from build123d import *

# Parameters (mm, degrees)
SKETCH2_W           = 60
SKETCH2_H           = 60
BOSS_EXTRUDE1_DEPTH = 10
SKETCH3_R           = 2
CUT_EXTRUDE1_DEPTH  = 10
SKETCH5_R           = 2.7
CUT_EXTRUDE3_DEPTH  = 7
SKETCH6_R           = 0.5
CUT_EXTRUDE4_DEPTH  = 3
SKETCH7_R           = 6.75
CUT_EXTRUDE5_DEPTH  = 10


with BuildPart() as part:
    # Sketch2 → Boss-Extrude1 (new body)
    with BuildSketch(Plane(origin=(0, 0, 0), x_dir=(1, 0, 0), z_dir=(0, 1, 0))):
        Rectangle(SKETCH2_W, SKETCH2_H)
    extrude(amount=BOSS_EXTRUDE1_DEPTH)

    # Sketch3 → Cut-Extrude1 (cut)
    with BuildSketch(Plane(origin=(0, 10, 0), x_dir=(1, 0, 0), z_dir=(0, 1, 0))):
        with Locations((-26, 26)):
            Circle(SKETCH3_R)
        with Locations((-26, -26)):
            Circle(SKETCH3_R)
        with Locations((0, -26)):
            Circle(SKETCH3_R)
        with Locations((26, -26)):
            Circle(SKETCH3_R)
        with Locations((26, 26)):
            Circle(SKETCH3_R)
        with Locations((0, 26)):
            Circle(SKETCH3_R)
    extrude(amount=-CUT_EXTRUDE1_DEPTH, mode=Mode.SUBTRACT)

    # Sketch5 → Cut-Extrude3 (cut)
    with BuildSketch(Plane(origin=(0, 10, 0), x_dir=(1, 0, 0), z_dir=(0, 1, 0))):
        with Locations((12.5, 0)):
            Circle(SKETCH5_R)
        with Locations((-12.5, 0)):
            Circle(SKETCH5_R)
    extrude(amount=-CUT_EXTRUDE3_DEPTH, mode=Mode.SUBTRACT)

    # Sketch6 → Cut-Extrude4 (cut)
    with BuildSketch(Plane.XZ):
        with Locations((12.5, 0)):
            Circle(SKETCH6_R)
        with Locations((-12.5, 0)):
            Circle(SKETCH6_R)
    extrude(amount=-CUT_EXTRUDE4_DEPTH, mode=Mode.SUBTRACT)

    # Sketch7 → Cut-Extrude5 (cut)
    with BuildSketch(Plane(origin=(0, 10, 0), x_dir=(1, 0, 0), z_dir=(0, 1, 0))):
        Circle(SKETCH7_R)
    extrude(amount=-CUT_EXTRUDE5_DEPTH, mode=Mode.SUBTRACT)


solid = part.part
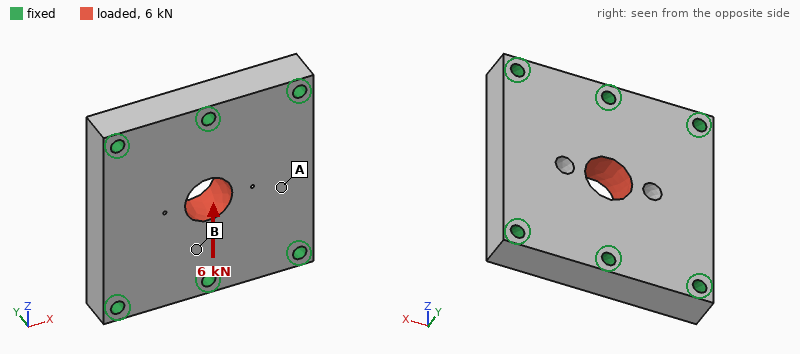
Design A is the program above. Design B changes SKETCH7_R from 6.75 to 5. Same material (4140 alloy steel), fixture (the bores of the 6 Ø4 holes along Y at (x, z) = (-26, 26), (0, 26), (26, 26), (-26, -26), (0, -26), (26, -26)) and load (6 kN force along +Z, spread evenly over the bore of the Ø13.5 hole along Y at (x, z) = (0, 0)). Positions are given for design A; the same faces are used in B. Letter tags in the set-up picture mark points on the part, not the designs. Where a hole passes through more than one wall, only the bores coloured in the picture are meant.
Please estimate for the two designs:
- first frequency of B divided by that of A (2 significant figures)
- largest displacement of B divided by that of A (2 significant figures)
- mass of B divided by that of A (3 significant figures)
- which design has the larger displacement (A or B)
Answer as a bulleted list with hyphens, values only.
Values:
- 0.99
- 1.2
- 1.02
- B
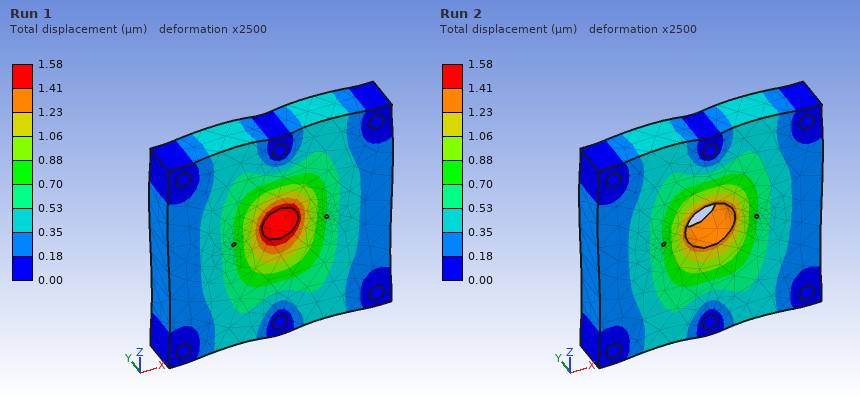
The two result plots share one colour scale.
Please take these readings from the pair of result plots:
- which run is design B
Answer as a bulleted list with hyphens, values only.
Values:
- Run 1
